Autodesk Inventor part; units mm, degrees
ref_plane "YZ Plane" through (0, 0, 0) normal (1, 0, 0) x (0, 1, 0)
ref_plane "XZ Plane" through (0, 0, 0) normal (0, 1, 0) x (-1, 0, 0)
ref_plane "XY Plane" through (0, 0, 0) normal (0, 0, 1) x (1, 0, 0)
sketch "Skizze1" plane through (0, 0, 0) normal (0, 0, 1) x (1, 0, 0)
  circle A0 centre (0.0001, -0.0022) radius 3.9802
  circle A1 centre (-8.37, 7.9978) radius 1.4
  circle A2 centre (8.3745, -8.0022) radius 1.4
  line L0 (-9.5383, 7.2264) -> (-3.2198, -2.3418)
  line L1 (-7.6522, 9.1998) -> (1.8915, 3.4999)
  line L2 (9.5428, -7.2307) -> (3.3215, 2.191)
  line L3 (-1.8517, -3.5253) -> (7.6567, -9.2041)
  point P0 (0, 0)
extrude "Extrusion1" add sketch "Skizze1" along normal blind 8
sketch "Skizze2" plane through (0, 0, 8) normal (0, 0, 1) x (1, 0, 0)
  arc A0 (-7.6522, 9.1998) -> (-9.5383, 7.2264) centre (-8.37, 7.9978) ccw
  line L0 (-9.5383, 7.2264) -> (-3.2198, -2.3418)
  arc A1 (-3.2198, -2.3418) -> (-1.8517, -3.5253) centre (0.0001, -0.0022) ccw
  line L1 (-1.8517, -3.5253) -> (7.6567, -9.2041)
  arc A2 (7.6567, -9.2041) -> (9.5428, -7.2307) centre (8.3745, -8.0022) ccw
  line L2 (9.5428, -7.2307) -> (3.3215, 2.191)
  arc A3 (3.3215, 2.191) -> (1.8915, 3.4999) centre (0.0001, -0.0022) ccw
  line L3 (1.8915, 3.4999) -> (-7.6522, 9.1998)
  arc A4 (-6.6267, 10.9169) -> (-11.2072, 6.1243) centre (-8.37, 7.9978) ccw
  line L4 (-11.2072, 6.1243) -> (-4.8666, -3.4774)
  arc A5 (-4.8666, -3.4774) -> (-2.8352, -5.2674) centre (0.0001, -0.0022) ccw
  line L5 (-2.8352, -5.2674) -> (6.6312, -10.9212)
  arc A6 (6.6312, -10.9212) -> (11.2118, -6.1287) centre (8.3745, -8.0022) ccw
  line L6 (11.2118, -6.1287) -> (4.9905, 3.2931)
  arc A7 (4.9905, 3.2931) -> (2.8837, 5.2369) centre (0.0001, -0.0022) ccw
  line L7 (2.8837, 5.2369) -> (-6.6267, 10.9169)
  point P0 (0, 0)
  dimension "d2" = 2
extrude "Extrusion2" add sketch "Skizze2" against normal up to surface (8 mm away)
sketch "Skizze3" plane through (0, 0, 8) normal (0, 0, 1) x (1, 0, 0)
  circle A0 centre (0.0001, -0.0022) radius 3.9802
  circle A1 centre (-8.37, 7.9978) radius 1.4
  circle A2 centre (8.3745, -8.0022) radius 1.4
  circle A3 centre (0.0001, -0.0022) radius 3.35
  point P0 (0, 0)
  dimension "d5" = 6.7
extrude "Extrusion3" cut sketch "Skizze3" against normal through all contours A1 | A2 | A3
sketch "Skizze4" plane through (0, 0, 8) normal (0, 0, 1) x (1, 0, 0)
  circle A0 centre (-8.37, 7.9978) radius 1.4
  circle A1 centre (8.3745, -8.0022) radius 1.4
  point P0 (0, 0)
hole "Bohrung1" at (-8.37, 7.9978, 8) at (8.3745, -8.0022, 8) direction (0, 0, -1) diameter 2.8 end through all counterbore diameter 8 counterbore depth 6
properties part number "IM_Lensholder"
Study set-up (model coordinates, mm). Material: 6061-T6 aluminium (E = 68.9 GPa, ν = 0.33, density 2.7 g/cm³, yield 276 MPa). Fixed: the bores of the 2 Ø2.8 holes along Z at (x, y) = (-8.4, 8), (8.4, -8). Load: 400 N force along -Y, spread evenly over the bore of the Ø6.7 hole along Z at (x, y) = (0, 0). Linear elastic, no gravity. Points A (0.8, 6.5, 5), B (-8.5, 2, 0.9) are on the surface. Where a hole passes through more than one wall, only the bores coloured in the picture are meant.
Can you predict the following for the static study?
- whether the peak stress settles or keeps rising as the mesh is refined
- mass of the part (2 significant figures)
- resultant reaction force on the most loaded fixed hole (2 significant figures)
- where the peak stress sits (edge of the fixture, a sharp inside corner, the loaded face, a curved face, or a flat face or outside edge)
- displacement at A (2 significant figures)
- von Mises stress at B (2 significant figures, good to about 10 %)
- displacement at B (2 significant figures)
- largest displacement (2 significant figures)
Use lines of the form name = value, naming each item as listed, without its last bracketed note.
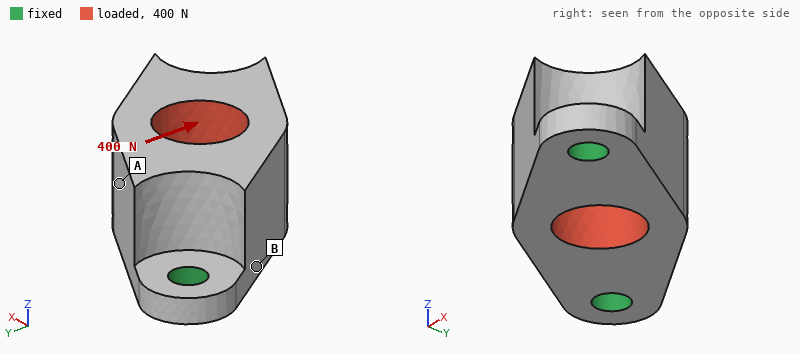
whether the peak stress settles or keeps rising as the mesh is refined = keeps rising
mass of the part = 3.4 g
resultant reaction force on the most loaded fixed hole = 200 N
where the peak stress sits = edge of the fixture
displacement at A = 14 µm
von Mises stress at B = 20 MPa
displacement at B = 6.8 µm
largest displacement = 19 µm
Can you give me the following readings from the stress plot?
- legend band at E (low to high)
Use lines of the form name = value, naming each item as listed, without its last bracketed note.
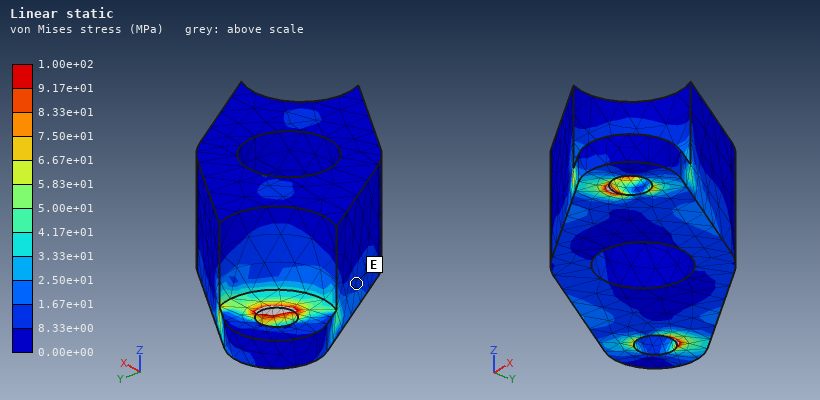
legend band at E = 8.33e+00 to 1.67e+01 MPa
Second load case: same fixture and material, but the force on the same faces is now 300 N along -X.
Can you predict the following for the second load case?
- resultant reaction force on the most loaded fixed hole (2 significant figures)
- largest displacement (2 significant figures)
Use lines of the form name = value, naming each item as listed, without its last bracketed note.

resultant reaction force on the most loaded fixed hole = 150 N
largest displacement = 13 µm
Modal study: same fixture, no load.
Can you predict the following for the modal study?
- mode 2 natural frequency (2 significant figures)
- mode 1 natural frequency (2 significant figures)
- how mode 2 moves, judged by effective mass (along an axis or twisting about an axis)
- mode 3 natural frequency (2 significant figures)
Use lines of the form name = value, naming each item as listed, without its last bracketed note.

mode 2 natural frequency = 25 kHz
mode 1 natural frequency = 13 kHz
how mode 2 moves, judged by effective mass = along Z
mode 3 natural frequency = 40 kHz
